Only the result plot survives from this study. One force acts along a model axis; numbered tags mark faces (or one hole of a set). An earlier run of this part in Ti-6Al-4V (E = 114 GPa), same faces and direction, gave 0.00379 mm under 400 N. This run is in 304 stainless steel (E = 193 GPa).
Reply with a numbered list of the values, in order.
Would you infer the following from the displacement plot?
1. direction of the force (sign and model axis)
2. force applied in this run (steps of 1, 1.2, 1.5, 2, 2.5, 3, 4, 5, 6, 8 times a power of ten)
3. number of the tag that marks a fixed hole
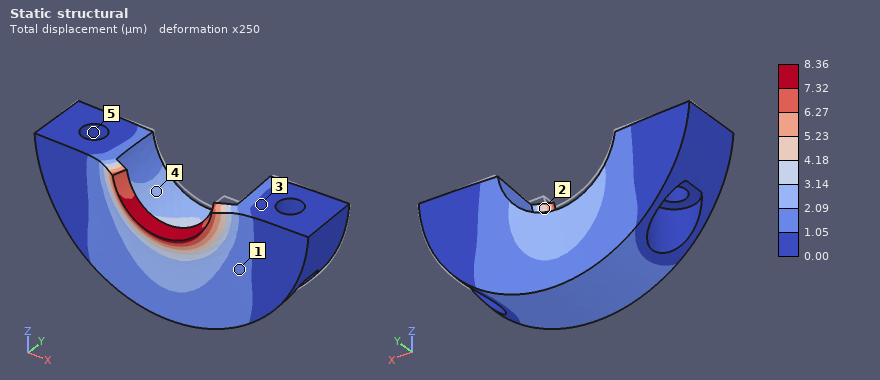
1. -Y
2. 1.5 kN
3. 5
